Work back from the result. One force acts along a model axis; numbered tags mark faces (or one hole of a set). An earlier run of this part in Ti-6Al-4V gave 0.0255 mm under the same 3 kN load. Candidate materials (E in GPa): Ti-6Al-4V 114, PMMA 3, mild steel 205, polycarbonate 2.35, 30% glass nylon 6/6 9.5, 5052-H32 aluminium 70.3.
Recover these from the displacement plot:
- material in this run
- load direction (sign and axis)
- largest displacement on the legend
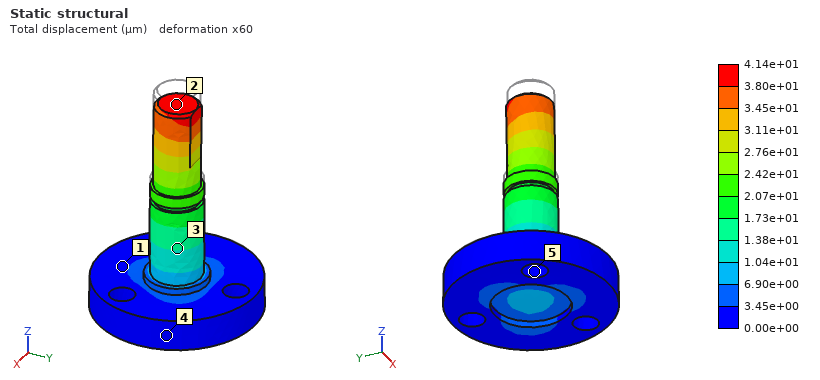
5052-H32 aluminium
-Z
4.14e+01 µm
